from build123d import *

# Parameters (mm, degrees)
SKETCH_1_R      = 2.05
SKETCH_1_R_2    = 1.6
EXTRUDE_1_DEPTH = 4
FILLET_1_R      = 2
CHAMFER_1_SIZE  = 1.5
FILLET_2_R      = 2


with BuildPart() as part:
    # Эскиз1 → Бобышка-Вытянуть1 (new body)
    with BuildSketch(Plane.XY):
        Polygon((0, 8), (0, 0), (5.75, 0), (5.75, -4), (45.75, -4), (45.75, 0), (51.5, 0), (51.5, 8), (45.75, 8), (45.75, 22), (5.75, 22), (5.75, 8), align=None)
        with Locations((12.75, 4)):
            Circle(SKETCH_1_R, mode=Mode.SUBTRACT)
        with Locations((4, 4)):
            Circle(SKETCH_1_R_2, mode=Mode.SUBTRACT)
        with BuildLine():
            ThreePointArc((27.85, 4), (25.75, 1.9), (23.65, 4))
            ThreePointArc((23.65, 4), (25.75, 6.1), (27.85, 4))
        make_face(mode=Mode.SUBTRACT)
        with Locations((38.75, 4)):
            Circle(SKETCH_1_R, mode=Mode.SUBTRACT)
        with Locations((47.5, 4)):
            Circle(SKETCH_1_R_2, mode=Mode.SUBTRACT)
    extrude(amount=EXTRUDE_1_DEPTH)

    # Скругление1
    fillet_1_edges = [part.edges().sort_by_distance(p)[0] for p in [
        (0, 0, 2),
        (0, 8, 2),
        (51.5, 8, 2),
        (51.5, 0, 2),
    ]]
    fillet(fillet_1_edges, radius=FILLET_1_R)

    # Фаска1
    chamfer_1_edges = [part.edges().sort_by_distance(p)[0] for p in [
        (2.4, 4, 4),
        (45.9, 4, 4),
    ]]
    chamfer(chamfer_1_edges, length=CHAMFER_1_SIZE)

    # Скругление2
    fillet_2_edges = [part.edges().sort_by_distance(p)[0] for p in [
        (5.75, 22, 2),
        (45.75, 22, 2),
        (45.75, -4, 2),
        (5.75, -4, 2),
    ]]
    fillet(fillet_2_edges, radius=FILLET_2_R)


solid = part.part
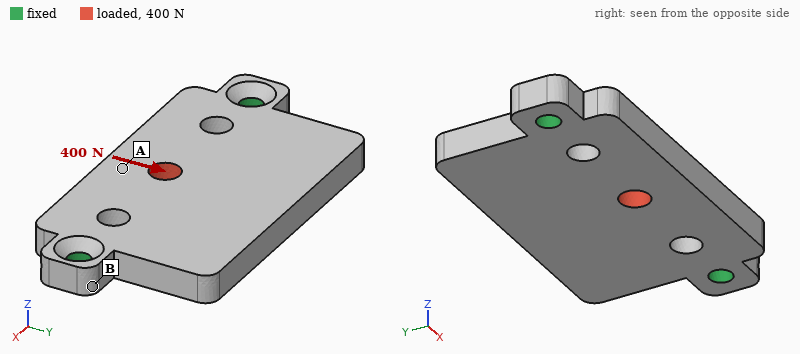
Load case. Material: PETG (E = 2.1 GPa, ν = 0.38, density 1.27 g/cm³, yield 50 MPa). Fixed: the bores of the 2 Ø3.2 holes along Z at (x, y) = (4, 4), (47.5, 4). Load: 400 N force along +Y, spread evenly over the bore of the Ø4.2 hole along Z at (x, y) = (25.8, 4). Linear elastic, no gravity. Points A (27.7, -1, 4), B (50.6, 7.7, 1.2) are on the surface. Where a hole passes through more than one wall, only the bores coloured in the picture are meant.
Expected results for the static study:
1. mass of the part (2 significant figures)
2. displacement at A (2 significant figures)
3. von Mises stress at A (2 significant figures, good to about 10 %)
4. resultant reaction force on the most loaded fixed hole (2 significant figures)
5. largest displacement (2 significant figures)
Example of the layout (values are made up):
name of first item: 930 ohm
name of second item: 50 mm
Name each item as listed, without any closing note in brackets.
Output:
mass of the part: 5.4 g
displacement at A: 0.15 mm
von Mises stress at A: 7.3 MPa
resultant reaction force on the most loaded fixed hole: 210 N
largest displacement: 0.17 mm
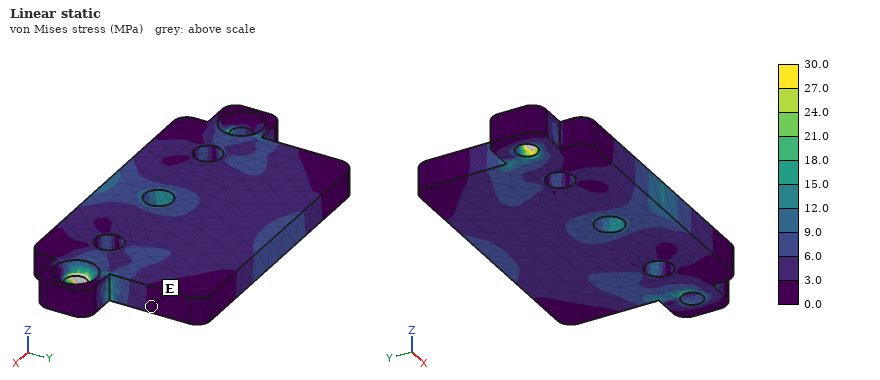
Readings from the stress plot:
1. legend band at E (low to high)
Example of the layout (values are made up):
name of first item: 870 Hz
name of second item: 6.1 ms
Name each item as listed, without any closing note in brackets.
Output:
legend band at E: 0.0 to 3.0 MPa
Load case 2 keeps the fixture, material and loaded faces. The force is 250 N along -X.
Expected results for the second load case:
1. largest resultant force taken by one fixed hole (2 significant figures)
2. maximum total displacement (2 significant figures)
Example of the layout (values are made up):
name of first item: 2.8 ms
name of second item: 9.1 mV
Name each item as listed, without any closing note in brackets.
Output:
largest resultant force taken by one fixed hole: 130 N
maximum total displacement: 40 µm
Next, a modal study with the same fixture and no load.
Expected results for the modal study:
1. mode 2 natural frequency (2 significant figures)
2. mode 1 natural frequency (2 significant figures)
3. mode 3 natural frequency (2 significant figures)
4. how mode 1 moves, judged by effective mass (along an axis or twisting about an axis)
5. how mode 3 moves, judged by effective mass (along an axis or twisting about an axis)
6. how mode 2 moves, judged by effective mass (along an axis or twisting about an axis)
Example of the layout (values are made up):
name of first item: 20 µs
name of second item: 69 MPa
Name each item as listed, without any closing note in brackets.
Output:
mode 2 natural frequency: 2300 Hz
mode 1 natural frequency: 1100 Hz
mode 3 natural frequency: 2900 Hz
how mode 1 moves, judged by effective mass: along Z
how mode 3 moves, judged by effective mass: twisting about Y
how mode 2 moves, judged by effective mass: along Z
